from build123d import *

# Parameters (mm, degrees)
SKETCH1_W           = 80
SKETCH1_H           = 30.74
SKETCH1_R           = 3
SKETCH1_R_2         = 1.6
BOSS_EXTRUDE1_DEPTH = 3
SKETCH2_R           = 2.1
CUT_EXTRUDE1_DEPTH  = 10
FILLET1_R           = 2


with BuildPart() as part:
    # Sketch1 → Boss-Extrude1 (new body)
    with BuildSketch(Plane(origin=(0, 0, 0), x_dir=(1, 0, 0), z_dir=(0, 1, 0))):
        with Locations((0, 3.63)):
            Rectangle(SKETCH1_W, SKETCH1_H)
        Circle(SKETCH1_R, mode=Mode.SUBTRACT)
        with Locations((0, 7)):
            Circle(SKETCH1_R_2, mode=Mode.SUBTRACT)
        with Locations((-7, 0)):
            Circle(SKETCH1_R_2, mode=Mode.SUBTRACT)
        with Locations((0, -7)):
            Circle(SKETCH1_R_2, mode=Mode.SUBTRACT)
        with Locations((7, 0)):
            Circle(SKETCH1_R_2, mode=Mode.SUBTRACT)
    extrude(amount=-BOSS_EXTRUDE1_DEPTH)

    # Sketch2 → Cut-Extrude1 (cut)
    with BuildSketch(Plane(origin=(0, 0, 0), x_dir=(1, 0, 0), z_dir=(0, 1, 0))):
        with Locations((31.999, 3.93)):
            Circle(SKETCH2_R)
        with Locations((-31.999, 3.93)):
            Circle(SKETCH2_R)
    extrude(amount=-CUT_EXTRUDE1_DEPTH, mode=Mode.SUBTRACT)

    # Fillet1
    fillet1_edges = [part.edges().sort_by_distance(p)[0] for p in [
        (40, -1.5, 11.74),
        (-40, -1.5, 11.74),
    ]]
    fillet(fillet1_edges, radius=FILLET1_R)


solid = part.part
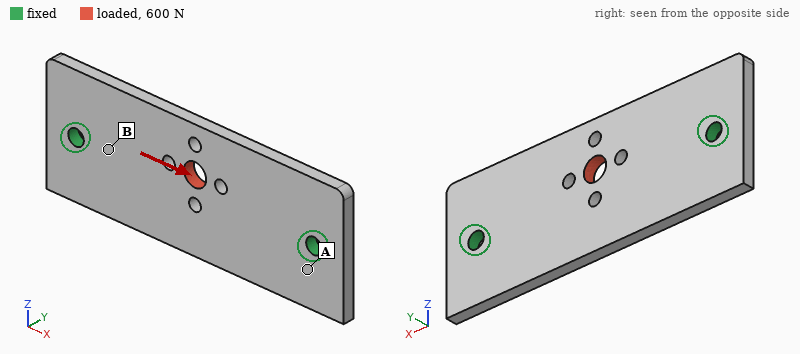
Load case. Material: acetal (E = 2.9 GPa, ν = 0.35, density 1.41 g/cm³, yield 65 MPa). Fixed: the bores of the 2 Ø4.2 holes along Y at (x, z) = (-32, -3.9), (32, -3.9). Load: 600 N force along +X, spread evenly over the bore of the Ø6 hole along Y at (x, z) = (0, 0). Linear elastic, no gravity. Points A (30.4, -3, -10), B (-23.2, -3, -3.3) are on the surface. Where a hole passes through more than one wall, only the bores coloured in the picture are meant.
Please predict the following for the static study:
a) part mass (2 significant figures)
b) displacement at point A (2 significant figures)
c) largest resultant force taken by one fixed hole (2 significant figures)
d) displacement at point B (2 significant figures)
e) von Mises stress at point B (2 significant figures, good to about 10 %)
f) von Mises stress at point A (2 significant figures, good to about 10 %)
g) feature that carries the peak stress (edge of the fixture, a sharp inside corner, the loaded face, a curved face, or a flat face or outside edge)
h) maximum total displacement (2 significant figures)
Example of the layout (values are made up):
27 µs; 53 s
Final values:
10 g; 14 µm; 300 N; 20 µm; 6.6 MPa; 2.6 MPa; a curved face; 81 µm
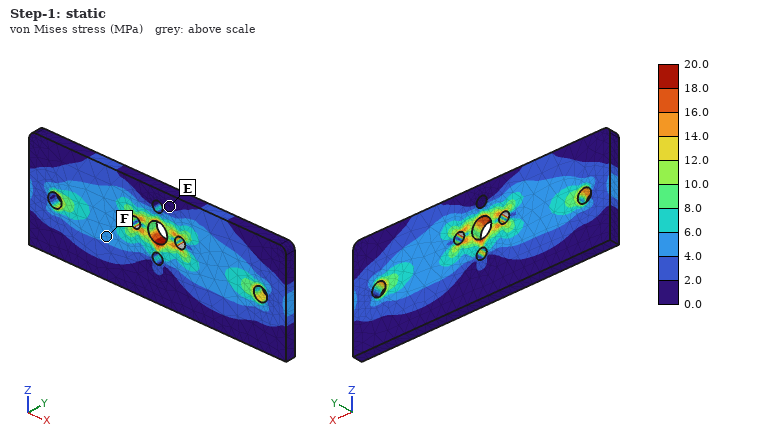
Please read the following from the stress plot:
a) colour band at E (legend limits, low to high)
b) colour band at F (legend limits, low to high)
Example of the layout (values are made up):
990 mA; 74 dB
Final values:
0.0 to 2.0 MPa; 4.0 to 6.0 MPa
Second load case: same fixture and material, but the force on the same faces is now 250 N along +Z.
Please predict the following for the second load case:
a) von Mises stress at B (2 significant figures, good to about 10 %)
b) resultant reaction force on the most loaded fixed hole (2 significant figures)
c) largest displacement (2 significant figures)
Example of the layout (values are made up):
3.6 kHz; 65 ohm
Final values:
3.5 MPa; 130 N; 0.12 mm
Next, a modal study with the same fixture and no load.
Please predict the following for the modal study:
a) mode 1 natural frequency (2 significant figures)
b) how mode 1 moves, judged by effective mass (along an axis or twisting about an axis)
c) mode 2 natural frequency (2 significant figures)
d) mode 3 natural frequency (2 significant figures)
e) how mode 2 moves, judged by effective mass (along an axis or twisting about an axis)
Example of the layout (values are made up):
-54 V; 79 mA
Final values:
1000 Hz; along Y; 1300 Hz; 2500 Hz; twisting about X
